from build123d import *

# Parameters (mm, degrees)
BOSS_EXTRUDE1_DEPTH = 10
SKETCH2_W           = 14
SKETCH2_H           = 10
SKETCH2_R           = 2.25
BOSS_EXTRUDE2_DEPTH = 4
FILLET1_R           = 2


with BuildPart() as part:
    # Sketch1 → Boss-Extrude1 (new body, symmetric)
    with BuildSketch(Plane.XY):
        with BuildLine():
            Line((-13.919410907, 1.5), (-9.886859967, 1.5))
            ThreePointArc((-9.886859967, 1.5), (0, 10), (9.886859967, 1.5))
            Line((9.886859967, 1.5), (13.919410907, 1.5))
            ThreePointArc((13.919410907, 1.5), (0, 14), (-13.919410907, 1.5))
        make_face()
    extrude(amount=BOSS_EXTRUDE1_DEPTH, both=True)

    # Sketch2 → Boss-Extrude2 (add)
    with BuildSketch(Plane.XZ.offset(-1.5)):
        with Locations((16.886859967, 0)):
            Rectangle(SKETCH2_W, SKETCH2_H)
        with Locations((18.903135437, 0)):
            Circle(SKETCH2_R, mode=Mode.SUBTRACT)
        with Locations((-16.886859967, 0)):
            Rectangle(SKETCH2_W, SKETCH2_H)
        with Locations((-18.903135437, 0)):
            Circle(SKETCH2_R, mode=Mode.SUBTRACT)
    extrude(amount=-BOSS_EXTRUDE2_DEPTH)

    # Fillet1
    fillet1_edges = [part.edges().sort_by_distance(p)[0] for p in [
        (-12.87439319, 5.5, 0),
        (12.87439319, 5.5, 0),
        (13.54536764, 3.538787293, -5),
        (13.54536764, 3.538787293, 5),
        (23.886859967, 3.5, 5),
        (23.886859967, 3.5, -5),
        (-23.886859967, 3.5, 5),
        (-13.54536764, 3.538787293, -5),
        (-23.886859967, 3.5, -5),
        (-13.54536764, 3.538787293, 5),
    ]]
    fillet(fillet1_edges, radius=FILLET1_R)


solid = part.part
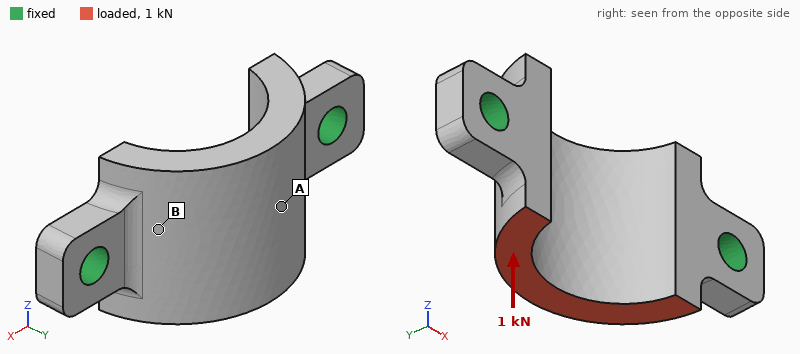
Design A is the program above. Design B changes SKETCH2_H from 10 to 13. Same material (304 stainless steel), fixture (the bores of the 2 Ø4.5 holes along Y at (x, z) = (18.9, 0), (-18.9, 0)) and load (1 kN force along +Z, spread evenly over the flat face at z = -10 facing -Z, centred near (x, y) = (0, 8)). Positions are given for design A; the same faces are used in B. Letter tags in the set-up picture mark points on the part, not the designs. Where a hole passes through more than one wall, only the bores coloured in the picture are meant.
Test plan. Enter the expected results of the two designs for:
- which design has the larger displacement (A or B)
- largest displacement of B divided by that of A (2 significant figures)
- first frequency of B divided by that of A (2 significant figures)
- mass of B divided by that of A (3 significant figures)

A
0.80
1.1
1.07
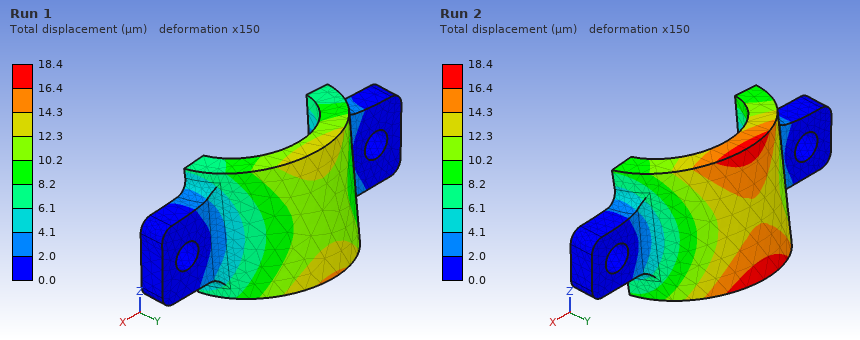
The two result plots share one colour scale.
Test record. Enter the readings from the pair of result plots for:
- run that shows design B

Run 1
